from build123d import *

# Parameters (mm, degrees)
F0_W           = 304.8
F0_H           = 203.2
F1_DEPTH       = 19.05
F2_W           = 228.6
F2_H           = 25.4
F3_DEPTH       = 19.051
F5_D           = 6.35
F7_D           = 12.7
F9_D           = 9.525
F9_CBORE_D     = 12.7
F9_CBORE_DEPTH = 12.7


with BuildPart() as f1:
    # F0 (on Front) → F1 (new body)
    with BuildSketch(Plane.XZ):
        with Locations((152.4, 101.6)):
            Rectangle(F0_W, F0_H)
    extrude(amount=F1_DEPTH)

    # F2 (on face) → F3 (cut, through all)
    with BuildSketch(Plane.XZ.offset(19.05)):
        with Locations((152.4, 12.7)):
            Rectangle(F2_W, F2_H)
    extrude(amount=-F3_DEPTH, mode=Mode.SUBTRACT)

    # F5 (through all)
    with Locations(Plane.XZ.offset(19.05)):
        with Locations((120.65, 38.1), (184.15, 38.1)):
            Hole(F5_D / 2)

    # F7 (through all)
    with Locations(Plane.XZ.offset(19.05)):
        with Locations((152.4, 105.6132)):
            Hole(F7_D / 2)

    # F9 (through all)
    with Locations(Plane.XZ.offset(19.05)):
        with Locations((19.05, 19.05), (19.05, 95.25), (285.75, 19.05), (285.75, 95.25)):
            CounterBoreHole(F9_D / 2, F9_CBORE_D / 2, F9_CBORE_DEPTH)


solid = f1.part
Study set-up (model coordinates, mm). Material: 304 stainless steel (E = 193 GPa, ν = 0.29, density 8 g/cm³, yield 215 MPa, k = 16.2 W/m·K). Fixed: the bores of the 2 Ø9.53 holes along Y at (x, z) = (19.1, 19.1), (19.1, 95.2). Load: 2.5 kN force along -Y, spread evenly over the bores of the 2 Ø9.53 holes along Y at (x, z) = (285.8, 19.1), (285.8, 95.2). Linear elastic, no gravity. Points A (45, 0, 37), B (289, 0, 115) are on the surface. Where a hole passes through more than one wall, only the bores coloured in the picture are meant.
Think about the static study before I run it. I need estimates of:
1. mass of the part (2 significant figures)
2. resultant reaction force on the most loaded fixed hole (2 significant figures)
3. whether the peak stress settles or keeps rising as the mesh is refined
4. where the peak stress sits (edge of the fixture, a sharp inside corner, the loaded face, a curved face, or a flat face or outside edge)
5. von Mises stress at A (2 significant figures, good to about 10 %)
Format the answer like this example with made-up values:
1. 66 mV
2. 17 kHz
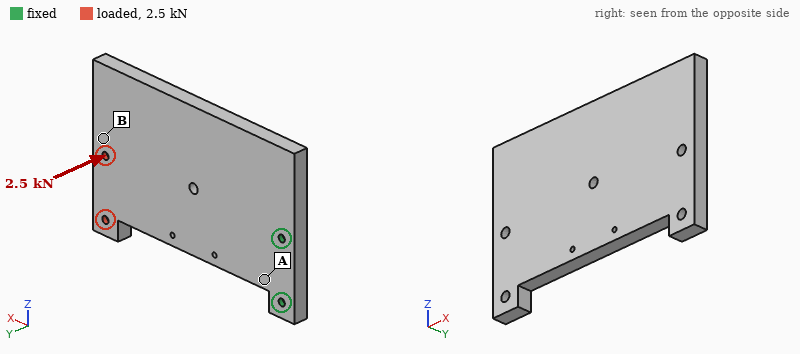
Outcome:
1. 8.5 kg
2. 3.4 kN
3. keeps rising
4. edge of the fixture
5. 98 MPa
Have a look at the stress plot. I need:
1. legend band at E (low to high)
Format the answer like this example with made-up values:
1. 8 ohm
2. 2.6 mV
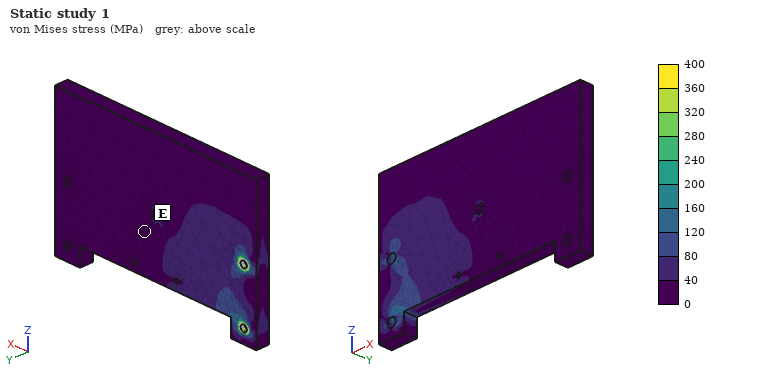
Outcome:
1. 0 to 40 MPa
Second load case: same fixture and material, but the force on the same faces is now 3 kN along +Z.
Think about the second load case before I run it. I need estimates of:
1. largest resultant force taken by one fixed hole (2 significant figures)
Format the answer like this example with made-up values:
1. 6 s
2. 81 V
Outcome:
1. 10 kN
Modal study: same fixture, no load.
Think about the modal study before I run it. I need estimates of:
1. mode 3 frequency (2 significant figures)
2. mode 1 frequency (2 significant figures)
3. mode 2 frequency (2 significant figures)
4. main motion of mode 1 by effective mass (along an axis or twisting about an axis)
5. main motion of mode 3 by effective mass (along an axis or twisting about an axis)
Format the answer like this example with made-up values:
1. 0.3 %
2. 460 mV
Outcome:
1. 550 Hz
2. 100 Hz
3. 430 Hz
4. along Y
5. along Z
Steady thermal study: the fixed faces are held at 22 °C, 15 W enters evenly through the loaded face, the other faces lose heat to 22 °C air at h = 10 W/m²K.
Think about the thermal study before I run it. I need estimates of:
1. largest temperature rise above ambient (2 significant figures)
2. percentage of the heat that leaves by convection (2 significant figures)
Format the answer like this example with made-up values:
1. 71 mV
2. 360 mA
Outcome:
1. 51 K
2. 91 %
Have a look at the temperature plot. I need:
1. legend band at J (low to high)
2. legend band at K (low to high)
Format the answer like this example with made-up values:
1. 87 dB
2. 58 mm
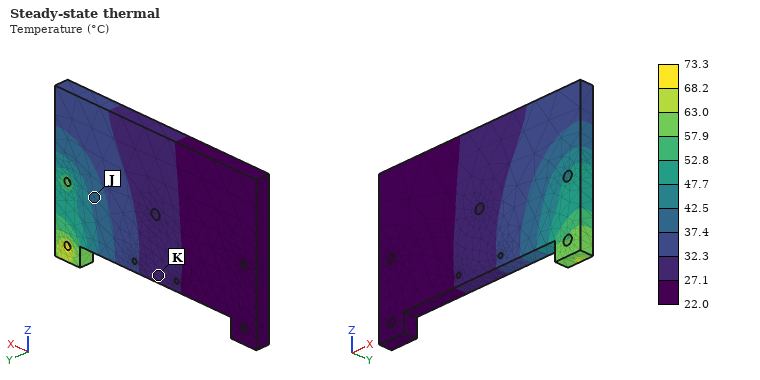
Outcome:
1. 37.4 to 42.5 °C
2. 27.1 to 32.3 °C
